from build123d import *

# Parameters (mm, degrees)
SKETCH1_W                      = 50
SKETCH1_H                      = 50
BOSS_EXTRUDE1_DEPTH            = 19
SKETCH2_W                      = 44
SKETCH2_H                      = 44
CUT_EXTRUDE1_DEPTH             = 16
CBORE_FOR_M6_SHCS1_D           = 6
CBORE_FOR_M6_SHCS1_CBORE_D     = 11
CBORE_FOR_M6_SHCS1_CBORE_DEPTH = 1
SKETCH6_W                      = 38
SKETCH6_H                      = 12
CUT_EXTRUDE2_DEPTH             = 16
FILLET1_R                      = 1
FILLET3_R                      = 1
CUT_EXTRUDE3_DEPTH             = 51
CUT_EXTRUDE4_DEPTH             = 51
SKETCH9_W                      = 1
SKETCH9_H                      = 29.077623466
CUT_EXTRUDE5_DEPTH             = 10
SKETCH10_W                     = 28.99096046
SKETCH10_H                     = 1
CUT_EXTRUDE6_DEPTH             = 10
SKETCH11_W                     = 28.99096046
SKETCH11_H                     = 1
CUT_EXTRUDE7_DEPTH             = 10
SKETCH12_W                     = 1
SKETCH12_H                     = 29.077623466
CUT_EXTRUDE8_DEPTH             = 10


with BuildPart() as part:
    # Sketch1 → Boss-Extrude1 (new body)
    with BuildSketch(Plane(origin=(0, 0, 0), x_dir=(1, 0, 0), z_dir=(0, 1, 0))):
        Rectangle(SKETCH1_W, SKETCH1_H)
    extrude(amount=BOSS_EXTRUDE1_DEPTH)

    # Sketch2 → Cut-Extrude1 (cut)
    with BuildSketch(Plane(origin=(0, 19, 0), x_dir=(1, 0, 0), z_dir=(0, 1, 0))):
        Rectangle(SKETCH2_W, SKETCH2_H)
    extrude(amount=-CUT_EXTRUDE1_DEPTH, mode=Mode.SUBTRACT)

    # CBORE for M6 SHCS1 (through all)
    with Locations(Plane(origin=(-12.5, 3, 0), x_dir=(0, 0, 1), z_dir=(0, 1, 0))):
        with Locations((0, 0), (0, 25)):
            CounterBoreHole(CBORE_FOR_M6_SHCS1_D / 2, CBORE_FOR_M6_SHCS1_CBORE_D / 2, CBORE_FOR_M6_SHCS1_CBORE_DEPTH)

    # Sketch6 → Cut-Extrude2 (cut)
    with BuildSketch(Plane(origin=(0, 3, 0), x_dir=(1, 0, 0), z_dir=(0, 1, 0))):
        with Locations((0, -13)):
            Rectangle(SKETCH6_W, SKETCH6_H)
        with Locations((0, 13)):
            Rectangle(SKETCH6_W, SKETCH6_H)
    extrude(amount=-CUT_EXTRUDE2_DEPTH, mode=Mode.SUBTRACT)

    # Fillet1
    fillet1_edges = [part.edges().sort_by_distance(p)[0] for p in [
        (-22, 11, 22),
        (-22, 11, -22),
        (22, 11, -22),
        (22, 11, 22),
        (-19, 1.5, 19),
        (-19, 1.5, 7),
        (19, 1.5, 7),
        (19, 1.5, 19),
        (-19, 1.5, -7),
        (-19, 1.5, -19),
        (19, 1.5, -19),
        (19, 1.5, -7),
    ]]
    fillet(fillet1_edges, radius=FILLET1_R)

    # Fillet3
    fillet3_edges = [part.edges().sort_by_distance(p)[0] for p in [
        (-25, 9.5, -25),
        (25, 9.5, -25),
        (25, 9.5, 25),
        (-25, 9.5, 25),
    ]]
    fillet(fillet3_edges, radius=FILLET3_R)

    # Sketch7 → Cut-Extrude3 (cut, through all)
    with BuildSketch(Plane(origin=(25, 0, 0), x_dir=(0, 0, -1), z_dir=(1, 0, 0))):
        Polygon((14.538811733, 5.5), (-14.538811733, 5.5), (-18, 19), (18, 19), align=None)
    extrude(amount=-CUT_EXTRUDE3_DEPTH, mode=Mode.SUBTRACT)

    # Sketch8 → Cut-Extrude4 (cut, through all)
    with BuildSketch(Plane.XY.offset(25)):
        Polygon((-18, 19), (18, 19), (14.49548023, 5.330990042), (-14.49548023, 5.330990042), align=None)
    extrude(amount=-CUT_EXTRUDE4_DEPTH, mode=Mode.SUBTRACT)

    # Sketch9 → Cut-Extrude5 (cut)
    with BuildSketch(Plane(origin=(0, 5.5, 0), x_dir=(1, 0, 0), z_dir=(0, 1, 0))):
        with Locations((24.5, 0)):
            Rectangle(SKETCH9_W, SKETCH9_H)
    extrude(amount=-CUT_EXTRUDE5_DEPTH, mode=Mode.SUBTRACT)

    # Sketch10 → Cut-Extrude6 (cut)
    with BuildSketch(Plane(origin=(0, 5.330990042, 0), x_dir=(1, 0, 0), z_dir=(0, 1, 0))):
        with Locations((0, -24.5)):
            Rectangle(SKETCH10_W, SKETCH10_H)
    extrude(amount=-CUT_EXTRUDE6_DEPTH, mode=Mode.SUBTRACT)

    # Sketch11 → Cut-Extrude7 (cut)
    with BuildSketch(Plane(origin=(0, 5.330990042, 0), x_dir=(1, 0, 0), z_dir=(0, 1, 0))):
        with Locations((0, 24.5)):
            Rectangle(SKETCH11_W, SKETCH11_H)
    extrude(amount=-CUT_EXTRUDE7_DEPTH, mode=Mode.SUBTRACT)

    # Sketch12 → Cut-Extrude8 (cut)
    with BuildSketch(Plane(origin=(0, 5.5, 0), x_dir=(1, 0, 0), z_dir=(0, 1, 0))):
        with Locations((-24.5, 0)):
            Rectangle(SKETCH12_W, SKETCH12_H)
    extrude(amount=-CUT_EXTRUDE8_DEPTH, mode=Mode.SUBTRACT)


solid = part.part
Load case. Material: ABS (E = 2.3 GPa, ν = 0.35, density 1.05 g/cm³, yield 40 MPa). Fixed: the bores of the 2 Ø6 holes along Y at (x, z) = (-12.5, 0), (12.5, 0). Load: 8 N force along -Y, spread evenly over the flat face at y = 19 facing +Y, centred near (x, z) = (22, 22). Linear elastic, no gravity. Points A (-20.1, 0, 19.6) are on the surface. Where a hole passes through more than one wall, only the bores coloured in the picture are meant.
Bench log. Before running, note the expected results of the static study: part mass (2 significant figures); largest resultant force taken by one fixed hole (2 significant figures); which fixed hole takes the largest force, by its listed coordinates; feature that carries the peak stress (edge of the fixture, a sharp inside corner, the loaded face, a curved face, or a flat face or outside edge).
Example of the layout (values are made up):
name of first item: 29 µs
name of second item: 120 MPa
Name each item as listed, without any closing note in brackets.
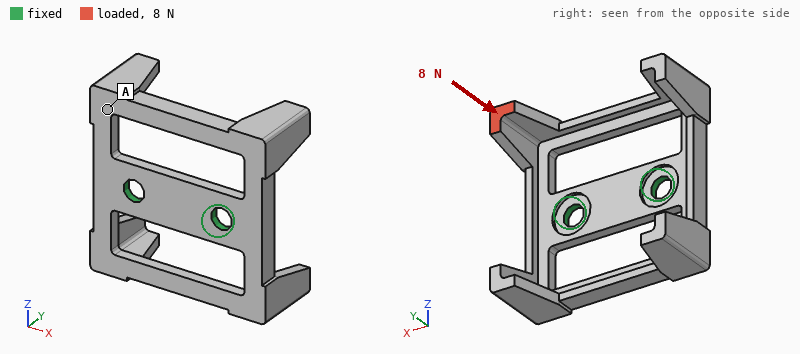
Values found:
part mass: 7.9 g
largest resultant force taken by one fixed hole: 8.9 N
which fixed hole takes the largest force, by its listed coordinates: (12.5, 0)
feature that carries the peak stress: a flat face or outside edge
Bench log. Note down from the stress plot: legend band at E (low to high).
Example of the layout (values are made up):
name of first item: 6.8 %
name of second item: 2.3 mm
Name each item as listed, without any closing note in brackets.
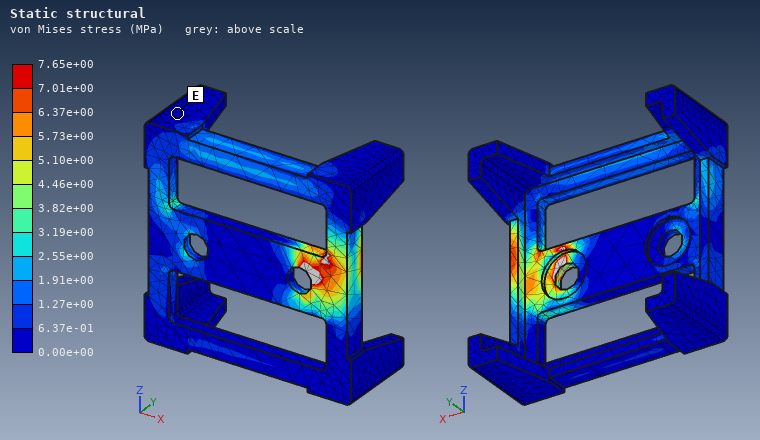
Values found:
legend band at E: 0.00e+00 to 6.37e-01 MPa
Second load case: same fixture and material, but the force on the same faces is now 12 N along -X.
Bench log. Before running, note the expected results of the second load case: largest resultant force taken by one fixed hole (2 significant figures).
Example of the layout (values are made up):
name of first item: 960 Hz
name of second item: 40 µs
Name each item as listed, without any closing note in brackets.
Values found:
largest resultant force taken by one fixed hole: 9.9 N
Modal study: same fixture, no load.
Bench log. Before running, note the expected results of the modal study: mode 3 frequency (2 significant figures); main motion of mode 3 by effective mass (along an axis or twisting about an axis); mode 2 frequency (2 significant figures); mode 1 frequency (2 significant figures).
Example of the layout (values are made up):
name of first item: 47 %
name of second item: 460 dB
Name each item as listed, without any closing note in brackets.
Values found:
mode 3 frequency: 670 Hz
main motion of mode 3 by effective mass: along Y
mode 2 frequency: 540 Hz
mode 1 frequency: 410 Hz
